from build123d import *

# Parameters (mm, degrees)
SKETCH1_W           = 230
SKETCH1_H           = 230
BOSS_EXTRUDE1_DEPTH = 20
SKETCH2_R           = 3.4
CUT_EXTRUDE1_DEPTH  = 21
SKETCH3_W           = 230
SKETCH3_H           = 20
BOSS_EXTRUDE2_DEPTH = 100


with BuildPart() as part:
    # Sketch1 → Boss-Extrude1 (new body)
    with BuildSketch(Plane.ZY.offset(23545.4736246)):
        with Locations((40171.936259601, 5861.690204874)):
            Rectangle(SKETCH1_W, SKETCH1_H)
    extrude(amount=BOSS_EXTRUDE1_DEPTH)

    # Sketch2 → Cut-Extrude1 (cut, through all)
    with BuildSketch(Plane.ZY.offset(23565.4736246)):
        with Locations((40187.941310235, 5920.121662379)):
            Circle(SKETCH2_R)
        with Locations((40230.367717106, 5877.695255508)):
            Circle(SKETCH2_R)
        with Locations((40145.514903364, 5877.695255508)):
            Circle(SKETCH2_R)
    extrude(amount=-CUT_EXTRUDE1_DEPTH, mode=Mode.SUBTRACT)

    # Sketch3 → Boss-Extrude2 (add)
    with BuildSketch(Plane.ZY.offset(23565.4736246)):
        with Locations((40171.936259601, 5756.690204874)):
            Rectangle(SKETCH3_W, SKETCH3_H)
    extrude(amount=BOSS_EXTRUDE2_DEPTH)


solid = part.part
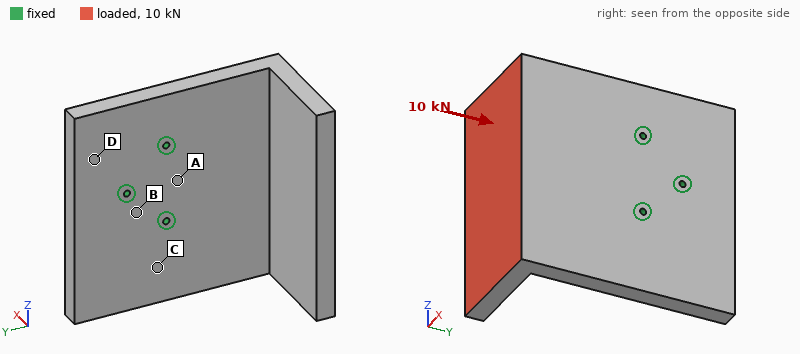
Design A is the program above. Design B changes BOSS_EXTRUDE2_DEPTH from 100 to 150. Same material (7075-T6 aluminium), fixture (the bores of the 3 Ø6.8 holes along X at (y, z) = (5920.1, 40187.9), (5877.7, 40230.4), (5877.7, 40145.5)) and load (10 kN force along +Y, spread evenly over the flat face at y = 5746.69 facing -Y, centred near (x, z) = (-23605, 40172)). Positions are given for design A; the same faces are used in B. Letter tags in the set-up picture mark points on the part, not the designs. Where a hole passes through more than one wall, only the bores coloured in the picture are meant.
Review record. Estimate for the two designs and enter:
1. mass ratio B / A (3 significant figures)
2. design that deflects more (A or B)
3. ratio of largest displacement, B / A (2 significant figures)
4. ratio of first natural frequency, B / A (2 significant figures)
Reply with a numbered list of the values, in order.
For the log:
1. 1.15
2. B
3. 2.1
4. 0.71
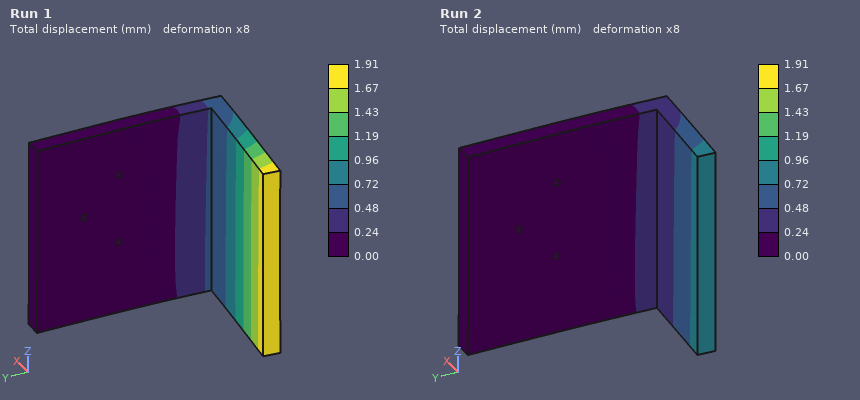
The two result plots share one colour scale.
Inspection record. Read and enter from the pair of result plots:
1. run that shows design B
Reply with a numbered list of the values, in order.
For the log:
1. Run 1
